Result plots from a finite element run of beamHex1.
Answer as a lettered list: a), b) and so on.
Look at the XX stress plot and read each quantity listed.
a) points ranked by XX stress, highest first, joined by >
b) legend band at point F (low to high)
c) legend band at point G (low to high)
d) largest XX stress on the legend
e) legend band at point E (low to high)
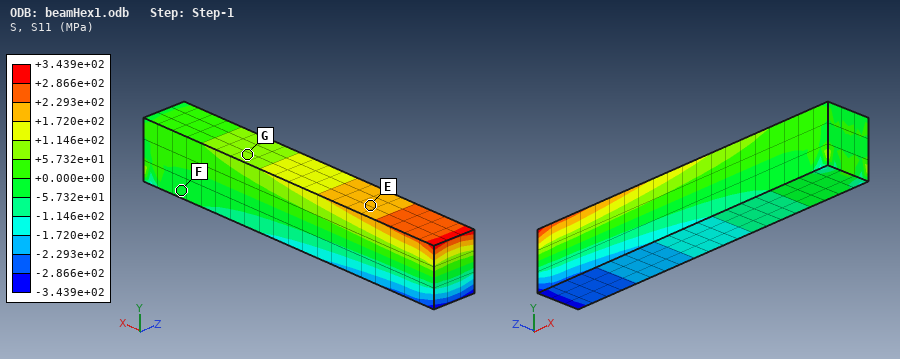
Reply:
a) E > G > F
b) -5.732e+01 to +0.000e+00 MPa
c) +5.732e+01 to +1.146e+02 MPa
d) +3.439e+02 MPa
e) +1.720e+02 to +2.293e+02 MPa
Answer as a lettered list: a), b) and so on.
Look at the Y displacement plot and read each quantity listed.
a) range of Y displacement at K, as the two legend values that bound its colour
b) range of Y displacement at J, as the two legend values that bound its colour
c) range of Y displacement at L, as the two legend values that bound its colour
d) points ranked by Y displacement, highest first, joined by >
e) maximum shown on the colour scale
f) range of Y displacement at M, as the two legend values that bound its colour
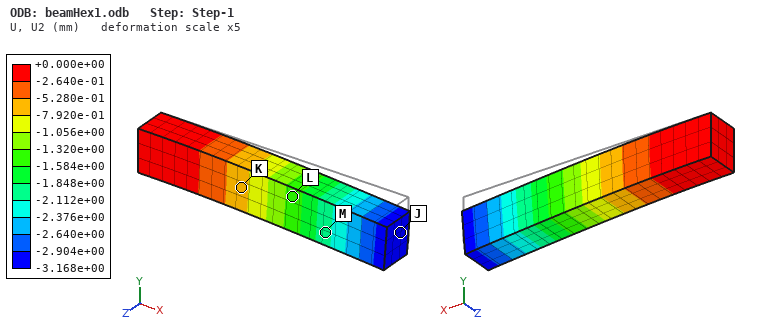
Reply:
a) -7.920e-01 to -5.280e-01 mm
b) -3.168e+00 to -2.904e+00 mm
c) -1.584e+00 to -1.320e+00 mm
d) K > L > M > J
e) +0.000e+00 mm
f) -2.112e+00 to -1.848e+00 mm
